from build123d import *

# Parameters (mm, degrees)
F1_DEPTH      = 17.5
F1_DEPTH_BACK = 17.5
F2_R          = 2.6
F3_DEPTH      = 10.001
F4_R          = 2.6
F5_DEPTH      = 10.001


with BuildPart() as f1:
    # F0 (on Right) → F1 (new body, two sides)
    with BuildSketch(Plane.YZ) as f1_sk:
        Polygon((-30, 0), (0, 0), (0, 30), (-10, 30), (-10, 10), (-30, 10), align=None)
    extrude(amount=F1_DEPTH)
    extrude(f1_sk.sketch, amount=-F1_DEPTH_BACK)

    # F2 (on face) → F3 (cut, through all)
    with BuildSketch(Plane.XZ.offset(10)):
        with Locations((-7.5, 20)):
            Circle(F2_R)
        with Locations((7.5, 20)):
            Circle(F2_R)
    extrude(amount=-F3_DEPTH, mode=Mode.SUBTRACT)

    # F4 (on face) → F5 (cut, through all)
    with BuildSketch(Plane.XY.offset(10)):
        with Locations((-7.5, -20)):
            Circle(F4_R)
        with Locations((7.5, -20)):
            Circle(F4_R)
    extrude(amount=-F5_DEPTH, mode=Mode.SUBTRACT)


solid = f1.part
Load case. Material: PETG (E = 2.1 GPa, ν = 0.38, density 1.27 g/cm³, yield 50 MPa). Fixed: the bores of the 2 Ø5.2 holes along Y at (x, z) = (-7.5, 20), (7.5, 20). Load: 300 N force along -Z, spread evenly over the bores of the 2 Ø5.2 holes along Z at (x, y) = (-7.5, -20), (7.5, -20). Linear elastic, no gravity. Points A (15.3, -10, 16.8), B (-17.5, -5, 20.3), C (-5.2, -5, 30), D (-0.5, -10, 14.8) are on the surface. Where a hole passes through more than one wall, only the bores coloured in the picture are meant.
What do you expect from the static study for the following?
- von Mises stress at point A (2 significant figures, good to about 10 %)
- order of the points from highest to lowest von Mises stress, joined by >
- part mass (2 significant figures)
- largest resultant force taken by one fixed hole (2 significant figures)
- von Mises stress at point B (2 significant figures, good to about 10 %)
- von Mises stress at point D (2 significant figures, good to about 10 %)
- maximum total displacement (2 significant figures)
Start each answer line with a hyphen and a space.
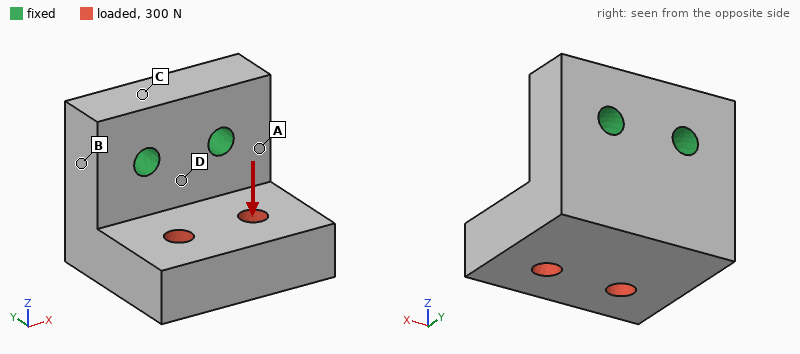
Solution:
- 4.8 MPa
- D > A > B > C
- 21 g
- 160 N
- 2.3 MPa
- 6.8 MPa
- 0.35 mm
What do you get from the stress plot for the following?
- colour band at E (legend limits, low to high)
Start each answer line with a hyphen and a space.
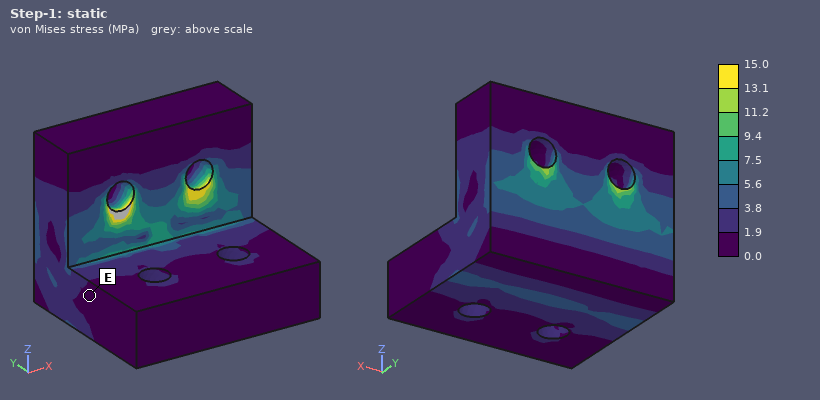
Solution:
- 0.0 to 1.9 MPa
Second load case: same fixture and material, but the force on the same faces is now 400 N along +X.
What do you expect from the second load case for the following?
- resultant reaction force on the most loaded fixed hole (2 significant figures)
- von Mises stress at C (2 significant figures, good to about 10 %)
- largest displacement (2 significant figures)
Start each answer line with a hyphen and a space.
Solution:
- 430 N
- 1.2 MPa
- 0.22 mm
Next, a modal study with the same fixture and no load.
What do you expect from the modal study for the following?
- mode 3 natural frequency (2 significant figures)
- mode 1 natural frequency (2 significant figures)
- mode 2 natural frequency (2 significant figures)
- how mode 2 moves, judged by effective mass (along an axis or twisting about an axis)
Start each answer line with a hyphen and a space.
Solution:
- 4000 Hz
- 1700 Hz
- 2500 Hz
- along X
